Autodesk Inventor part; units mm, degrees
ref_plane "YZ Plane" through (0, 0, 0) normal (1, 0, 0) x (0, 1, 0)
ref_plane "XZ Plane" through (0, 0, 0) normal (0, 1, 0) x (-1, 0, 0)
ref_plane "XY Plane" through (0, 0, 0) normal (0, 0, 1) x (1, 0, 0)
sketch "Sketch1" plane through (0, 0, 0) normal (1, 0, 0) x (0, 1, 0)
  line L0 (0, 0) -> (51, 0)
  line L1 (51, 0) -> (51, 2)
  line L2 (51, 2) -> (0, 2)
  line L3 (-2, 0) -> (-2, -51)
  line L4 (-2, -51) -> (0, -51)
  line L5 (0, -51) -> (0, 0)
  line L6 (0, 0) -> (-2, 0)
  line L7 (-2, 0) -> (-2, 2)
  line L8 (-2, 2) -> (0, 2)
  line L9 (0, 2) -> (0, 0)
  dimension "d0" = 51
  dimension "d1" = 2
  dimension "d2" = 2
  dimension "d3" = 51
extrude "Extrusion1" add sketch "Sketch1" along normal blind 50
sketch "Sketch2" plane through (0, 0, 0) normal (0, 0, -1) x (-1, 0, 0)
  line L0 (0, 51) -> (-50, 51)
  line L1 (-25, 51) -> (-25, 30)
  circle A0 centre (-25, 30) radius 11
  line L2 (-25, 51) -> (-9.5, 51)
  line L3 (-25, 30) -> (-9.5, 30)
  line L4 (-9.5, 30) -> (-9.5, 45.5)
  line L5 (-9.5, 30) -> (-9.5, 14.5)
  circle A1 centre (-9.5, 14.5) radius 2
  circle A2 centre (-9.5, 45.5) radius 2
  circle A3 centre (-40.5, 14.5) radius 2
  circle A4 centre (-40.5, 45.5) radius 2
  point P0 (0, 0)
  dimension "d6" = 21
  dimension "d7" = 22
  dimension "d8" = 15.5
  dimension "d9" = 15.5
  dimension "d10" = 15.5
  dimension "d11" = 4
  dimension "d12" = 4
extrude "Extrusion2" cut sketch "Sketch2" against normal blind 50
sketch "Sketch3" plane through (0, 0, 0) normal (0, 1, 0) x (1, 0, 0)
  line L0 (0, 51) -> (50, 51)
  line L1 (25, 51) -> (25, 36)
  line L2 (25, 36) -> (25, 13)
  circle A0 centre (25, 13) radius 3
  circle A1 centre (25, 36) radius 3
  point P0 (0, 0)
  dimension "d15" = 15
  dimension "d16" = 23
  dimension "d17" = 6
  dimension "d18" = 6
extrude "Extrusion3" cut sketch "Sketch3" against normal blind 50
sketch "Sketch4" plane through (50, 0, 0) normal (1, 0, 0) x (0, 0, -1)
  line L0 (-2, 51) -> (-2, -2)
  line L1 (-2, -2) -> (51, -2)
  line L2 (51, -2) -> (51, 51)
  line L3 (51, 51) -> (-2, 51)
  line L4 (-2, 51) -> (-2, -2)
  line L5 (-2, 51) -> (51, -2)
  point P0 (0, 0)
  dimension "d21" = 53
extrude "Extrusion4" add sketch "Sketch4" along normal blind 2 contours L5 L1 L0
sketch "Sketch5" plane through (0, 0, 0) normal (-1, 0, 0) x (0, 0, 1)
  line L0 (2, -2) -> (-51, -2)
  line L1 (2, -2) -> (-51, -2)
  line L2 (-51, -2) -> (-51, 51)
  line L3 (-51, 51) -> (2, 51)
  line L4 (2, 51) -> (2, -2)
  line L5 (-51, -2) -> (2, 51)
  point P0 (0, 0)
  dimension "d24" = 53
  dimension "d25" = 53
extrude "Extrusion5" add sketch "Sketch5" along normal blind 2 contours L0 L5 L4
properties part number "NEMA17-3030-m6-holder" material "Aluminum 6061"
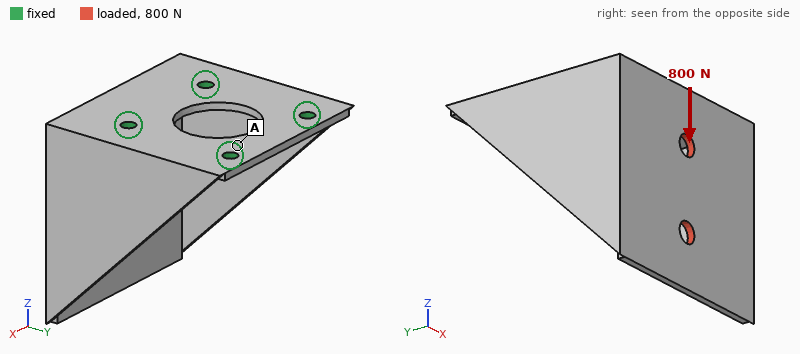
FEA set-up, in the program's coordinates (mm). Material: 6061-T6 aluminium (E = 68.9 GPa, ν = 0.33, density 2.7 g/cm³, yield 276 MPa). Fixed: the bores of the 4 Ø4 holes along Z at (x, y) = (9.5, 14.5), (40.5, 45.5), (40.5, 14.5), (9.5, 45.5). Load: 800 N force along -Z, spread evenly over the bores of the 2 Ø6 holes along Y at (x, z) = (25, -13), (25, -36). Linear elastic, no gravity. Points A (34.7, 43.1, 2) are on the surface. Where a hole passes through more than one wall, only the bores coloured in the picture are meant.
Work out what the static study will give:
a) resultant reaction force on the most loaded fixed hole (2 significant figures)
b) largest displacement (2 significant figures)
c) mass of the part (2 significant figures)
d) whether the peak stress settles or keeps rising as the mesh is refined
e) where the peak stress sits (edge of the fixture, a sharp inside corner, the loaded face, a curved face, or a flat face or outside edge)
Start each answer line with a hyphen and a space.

- 550 N
- 0.21 mm
- 41 g
- keeps rising
- edge of the fixture
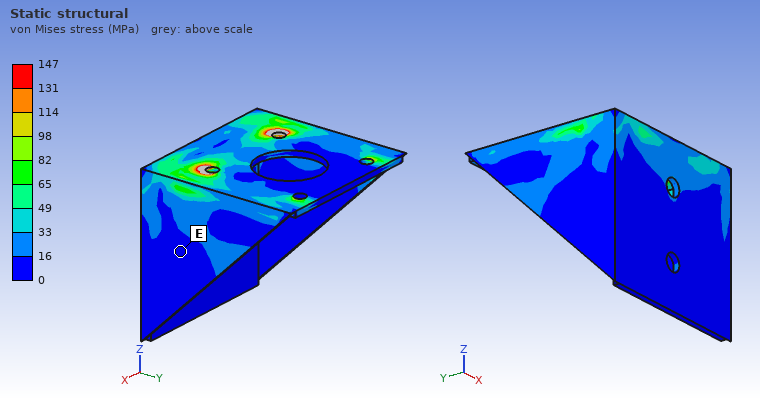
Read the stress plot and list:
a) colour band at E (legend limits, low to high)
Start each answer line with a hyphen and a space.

- 0 to 16 MPa
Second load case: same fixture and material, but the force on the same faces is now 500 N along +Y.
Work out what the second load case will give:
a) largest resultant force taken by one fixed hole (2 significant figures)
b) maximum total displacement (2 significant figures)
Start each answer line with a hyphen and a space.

- 290 N
- 0.51 mm
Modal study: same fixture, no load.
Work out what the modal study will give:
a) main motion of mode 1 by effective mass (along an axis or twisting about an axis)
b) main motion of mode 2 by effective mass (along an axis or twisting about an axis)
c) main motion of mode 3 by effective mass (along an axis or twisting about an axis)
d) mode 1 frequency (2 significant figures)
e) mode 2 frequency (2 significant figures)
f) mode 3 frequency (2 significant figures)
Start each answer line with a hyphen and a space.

- along X
- along Y
- along Z
- 1500 Hz
- 1700 Hz
- 2900 Hz
